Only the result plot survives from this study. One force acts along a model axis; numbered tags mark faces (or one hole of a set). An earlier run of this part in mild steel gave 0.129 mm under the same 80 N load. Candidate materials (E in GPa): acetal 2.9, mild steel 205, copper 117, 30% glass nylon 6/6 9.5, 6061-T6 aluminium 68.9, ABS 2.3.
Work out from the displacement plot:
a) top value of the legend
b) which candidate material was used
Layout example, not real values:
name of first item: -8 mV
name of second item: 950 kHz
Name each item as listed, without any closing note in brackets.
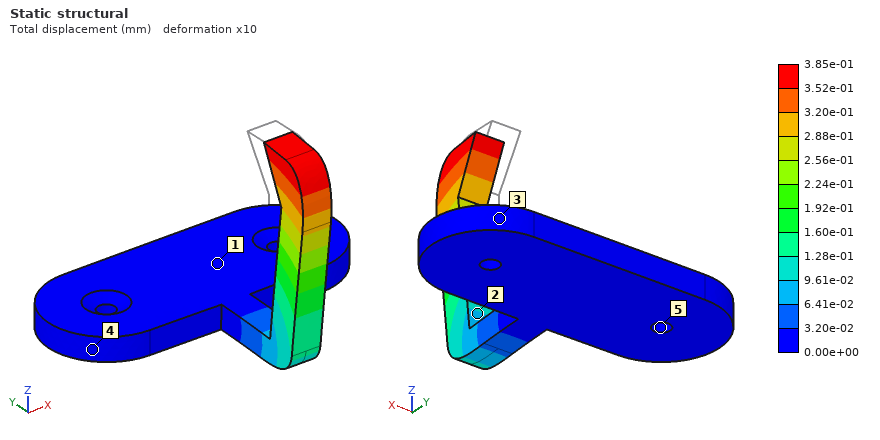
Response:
top value of the legend: 3.85e-01 mm
which candidate material was used: 6061-T6 aluminium
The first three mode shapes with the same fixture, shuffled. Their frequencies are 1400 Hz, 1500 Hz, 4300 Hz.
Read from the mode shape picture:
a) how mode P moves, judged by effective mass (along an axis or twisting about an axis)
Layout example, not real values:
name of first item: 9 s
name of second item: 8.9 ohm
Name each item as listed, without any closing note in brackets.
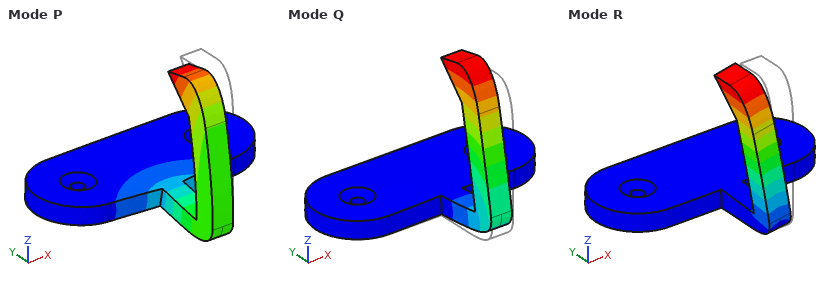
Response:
how mode P moves, judged by effective mass: along Z
